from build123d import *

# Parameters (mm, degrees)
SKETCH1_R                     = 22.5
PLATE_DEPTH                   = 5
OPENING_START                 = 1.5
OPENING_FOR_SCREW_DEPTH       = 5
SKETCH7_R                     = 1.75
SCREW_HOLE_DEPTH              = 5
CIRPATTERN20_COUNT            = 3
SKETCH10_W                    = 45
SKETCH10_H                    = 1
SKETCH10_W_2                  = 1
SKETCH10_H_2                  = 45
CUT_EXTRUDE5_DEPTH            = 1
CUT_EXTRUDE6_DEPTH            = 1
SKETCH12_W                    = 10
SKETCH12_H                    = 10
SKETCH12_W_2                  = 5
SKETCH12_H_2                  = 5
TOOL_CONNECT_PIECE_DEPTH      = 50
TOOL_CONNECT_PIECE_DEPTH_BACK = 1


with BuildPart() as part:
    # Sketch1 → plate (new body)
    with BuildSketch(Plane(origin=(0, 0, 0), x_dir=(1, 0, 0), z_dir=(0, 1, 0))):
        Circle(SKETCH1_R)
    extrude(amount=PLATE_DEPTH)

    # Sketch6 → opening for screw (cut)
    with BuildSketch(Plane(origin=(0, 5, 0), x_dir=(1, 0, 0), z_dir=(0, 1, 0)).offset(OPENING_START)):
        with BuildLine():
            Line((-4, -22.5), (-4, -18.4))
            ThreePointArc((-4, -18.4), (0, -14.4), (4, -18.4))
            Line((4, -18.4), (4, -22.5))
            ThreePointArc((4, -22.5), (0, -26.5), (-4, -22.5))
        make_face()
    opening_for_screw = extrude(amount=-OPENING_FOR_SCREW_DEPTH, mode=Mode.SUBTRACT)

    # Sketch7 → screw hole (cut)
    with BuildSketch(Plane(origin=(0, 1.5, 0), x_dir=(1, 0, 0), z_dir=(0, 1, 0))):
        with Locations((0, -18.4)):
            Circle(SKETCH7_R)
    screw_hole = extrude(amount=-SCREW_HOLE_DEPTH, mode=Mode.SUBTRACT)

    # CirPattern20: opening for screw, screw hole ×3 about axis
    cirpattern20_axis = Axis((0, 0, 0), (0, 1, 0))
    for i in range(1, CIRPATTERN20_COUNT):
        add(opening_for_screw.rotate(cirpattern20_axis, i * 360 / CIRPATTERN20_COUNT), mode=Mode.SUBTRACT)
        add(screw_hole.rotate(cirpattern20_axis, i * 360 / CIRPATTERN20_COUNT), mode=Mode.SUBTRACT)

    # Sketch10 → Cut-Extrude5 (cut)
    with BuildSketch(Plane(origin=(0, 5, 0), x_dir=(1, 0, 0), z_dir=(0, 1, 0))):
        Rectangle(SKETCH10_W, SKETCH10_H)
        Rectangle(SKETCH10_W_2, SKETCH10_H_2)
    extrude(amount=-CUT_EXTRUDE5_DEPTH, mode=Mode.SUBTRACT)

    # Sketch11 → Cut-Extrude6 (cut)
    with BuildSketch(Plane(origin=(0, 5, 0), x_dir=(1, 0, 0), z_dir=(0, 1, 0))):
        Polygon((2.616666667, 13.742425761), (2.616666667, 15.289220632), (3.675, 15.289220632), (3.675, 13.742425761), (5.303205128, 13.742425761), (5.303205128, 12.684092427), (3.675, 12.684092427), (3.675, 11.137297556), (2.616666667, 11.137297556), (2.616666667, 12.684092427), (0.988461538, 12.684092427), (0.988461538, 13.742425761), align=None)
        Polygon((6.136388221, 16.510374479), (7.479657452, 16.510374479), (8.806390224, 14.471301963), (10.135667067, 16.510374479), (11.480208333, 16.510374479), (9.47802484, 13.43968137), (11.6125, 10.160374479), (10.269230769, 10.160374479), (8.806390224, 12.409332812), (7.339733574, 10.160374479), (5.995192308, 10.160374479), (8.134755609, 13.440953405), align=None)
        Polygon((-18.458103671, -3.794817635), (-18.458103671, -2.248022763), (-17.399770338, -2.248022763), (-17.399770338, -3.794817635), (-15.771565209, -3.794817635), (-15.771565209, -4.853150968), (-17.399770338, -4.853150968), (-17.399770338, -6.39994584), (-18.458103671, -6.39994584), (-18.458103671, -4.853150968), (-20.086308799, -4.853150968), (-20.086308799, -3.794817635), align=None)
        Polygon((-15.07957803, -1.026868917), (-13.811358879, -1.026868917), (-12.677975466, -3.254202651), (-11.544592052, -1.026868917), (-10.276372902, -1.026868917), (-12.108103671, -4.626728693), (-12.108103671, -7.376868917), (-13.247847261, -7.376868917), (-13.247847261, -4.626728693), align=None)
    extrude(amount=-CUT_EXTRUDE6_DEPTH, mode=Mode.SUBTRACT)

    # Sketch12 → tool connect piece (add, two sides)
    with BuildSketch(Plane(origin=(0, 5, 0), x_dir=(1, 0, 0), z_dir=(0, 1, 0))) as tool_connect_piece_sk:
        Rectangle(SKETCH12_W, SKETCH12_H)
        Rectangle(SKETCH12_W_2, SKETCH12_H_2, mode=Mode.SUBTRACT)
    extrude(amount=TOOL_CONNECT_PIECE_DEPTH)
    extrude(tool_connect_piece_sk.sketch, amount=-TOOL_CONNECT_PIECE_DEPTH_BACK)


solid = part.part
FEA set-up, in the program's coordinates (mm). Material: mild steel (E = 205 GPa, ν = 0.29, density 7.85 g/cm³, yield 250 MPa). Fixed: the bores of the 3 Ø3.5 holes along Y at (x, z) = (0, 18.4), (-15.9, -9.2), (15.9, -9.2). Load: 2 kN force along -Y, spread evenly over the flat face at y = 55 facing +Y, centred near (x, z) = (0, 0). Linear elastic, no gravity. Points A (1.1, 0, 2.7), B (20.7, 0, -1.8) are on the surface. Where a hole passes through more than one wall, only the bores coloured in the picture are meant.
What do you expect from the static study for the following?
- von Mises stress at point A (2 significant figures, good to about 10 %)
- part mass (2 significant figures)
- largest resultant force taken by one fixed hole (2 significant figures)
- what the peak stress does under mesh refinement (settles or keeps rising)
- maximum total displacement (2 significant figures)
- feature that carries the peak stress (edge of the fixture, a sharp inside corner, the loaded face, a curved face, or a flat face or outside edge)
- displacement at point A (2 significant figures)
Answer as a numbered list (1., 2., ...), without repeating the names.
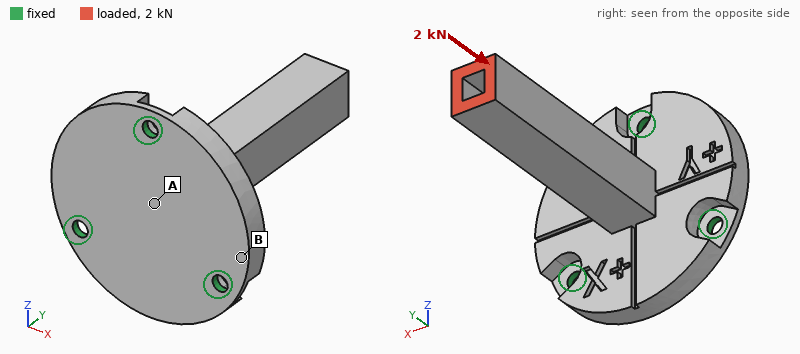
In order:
1. 45 MPa
2. 86 g
3. 960 N
4. keeps rising
5. 18 µm
6. edge of the fixture
7. 12 µm
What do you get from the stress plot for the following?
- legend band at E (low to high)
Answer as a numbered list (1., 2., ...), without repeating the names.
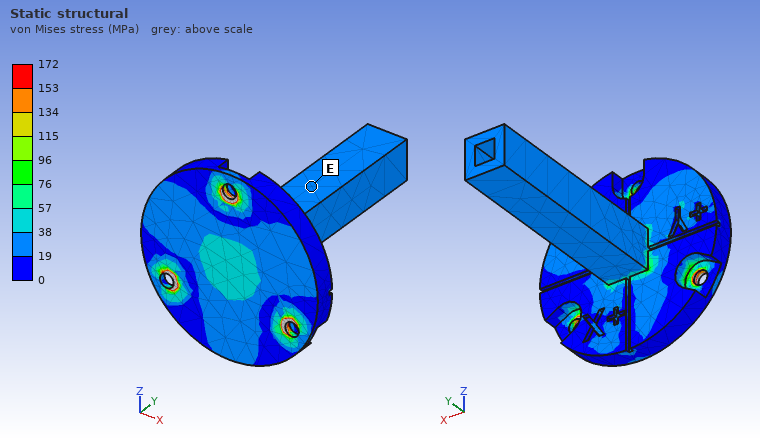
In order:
1. 19 to 38 MPa
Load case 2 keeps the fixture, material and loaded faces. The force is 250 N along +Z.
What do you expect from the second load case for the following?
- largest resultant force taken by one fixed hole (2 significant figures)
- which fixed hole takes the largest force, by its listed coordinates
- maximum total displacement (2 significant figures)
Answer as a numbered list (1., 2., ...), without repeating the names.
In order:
1. 650 N
2. (0, 18.4)
3. 0.11 mm
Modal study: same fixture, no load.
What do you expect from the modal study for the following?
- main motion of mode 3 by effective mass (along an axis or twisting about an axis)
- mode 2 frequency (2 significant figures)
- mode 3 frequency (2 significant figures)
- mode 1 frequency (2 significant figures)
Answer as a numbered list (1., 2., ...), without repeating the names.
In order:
1. along Y
2. 2600 Hz
3. 8900 Hz
4. 2600 Hz
